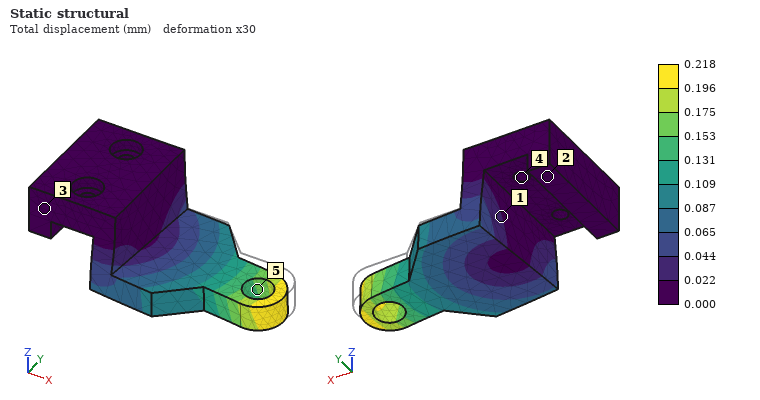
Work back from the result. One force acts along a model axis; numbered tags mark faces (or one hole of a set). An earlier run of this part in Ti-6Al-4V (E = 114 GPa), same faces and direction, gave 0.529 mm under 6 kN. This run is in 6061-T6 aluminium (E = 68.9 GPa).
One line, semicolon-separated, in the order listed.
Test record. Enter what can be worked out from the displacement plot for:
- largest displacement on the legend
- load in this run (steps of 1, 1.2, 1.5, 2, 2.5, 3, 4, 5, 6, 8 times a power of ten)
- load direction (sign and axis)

0.218 mm; 1.5 kN; -Y
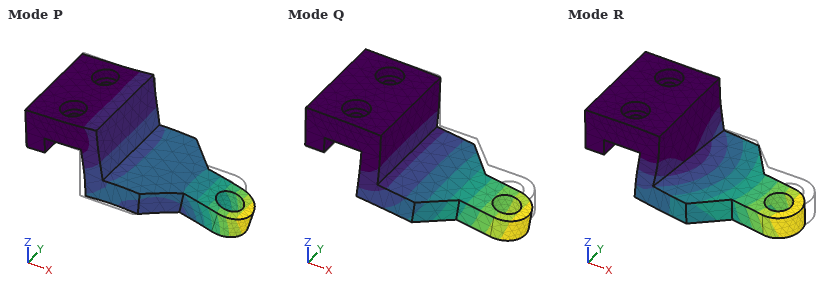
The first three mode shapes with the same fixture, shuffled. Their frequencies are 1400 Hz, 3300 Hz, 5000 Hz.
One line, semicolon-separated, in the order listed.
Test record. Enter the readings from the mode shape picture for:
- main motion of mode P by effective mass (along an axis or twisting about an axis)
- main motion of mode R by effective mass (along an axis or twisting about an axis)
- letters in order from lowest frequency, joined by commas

along X; along Y; Q, R, P
